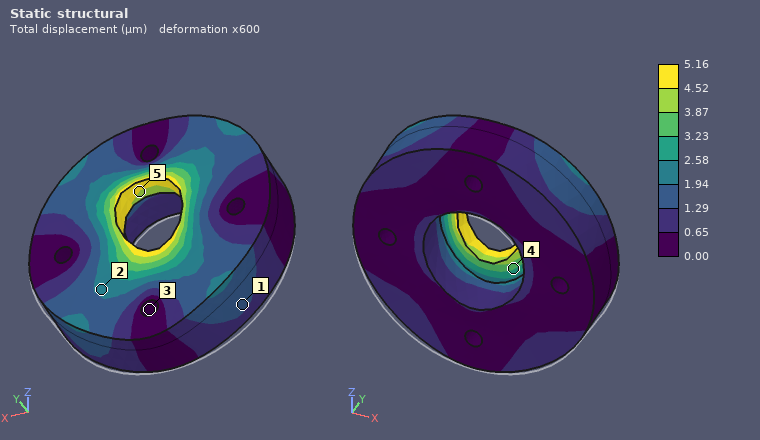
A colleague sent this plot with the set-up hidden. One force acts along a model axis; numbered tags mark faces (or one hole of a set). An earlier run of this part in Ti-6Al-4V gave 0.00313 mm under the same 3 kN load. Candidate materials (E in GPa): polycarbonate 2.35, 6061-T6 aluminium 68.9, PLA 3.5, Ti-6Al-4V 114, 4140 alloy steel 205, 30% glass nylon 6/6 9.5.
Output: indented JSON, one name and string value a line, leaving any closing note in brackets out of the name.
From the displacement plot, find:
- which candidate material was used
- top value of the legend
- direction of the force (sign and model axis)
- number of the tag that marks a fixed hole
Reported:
{
  "which candidate material was used": "6061-T6 aluminium",
  "top value of the legend": "5.16 µm",
  "direction of the force": "+Z",
  "number of the tag that marks a fixed hole": "3"
}
